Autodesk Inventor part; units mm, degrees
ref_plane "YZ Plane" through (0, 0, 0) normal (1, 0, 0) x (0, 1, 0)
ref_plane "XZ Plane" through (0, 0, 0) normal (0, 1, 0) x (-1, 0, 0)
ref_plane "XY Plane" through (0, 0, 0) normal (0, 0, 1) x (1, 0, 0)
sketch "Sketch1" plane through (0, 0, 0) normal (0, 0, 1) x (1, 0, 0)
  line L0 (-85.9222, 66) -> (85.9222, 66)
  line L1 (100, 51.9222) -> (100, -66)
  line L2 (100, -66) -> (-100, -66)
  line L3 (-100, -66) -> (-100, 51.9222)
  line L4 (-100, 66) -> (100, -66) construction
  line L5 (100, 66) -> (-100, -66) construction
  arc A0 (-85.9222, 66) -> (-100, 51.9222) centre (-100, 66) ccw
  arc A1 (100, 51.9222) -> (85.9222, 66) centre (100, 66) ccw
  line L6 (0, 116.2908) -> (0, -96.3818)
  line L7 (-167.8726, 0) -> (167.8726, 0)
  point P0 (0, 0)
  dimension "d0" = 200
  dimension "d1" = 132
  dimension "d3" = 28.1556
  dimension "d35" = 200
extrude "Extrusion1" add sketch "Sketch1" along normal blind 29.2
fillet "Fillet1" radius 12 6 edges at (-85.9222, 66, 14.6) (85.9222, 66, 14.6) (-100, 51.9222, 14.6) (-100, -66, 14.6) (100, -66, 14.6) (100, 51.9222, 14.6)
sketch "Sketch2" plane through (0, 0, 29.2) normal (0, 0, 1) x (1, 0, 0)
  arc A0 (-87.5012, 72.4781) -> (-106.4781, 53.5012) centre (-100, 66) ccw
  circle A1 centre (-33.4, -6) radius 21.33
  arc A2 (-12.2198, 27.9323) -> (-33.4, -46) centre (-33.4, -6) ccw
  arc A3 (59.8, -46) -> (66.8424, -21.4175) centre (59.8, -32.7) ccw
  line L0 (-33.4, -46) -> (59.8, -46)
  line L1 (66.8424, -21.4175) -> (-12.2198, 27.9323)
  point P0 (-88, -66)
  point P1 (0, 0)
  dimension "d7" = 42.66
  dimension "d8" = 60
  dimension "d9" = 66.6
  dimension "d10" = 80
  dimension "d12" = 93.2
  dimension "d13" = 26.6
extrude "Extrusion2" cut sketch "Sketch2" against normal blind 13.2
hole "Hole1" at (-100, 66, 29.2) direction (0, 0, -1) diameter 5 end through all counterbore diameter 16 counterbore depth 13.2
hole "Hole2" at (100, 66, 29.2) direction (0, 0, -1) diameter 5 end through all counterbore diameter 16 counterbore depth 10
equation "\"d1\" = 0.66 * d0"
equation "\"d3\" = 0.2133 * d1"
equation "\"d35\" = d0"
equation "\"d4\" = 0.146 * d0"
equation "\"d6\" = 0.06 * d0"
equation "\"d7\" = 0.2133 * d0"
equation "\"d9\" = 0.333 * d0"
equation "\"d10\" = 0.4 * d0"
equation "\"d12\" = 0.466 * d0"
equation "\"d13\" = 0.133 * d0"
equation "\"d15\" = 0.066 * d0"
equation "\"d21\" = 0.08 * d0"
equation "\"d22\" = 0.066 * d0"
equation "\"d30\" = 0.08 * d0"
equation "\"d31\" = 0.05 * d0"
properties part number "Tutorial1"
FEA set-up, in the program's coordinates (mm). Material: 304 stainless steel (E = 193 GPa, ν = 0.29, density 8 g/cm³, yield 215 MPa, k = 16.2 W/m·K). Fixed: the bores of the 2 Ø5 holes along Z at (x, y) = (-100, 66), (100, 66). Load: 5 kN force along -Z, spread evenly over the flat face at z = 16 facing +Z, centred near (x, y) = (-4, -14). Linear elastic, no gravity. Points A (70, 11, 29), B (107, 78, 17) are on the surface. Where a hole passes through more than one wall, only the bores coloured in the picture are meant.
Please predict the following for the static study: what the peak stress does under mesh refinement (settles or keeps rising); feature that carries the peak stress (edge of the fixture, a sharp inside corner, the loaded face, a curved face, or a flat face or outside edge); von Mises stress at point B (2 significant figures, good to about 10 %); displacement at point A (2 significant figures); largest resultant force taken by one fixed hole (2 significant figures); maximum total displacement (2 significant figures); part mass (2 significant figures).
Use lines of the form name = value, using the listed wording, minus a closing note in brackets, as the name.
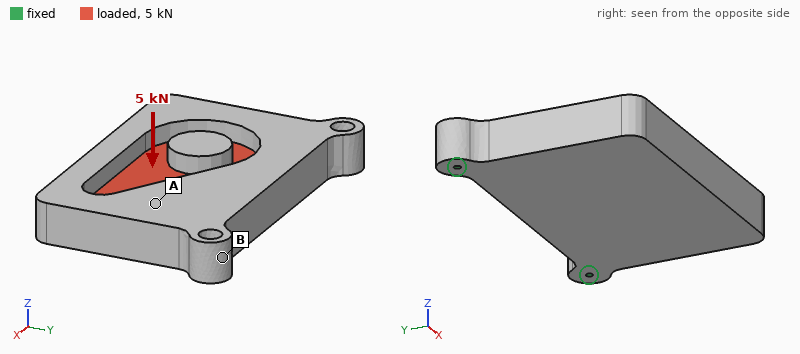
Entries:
what the peak stress does under mesh refinement = keeps rising
feature that carries the peak stress = edge of the fixture
von Mises stress at point B = 33 MPa
displacement at point A = 0.075 mm
largest resultant force taken by one fixed hole = 2.7 kN
maximum total displacement = 0.20 mm
part mass = 5.6 kg
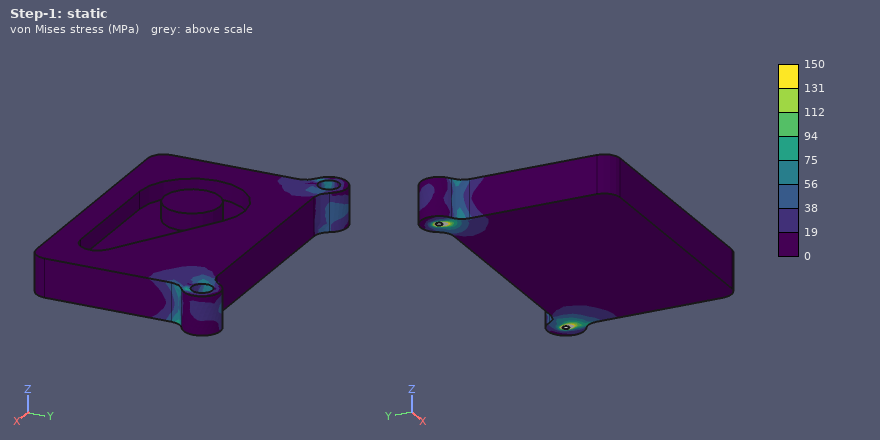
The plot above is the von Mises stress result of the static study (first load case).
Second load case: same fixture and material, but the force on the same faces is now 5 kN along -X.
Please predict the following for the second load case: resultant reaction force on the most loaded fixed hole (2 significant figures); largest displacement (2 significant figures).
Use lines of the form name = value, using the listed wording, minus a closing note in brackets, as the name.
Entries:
resultant reaction force on the most loaded fixed hole = 3.2 kN
largest displacement = 4.6 µm
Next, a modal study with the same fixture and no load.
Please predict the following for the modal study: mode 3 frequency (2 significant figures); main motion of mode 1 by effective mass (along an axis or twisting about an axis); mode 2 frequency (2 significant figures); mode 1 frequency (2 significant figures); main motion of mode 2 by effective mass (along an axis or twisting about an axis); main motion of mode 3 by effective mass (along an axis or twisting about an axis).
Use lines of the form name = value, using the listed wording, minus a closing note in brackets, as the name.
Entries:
mode 3 frequency = 2300 Hz
main motion of mode 1 by effective mass = along Z
mode 2 frequency = 1500 Hz
mode 1 frequency = 480 Hz
main motion of mode 2 by effective mass = twisting about Y
main motion of mode 3 by effective mass = along Z
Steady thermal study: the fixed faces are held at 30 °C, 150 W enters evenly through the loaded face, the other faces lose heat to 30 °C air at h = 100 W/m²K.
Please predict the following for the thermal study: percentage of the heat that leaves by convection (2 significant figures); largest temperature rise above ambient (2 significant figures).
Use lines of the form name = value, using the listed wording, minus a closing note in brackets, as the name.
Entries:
percentage of the heat that leaves by convection = 96 %
largest temperature rise above ambient = 64 K
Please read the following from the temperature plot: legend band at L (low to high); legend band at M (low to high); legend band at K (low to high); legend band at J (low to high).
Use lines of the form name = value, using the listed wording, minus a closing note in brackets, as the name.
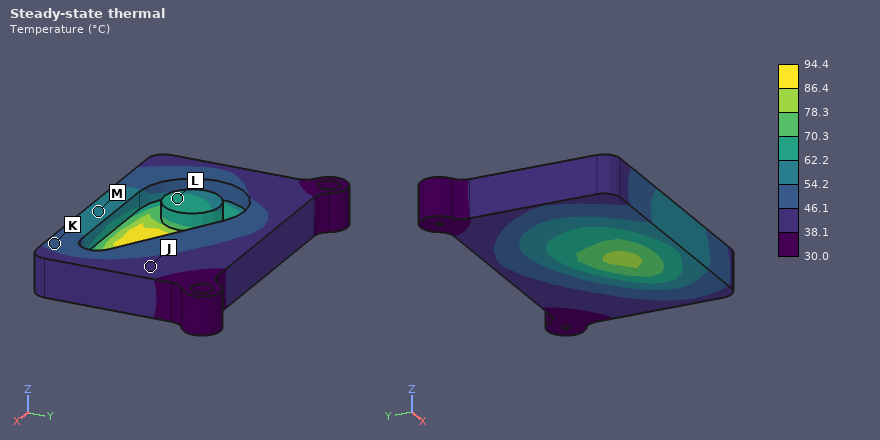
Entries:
legend band at L = 62.2 to 70.3 °C
legend band at M = 54.2 to 62.2 °C
legend band at K = 46.1 to 54.2 °C
legend band at J = 38.1 to 46.1 °C
